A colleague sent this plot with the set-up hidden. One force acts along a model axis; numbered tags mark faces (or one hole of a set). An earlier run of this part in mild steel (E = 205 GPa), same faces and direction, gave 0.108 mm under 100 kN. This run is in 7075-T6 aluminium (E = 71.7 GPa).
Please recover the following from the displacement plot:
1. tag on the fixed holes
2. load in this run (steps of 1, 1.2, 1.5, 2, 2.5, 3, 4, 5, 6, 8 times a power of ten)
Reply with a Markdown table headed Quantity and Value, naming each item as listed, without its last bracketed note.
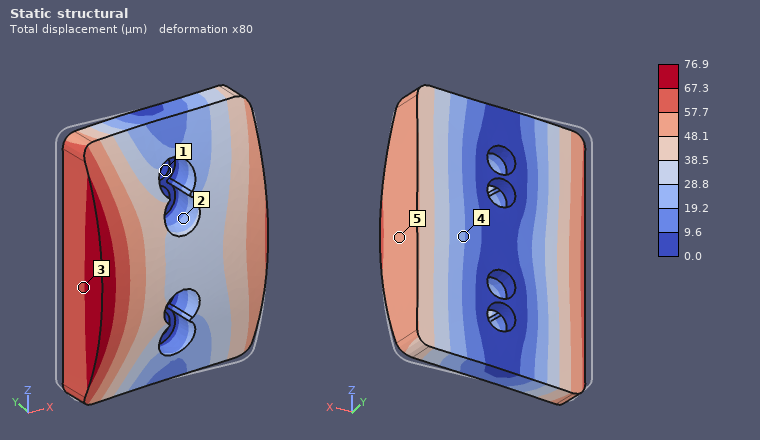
| Quantity | Value |
|---|---|
| tag on the fixed holes | 1 |
| load in this run | 25 kN |
